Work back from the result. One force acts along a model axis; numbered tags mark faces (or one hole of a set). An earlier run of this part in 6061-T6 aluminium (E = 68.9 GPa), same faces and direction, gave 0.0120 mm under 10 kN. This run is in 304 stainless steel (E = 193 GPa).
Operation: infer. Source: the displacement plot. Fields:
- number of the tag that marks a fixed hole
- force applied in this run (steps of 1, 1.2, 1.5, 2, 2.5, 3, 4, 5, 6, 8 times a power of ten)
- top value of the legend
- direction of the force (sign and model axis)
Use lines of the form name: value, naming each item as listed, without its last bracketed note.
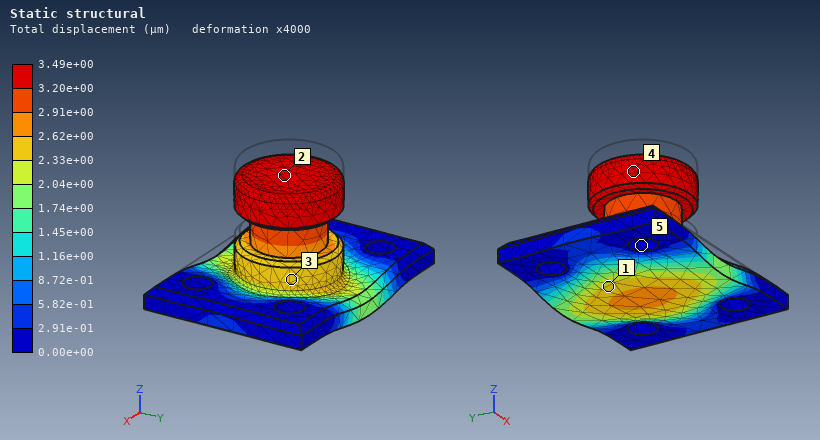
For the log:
number of the tag that marks a fixed hole: 5
force applied in this run: 8 kN
top value of the legend: 3.49e+00 µm
direction of the force: -Z
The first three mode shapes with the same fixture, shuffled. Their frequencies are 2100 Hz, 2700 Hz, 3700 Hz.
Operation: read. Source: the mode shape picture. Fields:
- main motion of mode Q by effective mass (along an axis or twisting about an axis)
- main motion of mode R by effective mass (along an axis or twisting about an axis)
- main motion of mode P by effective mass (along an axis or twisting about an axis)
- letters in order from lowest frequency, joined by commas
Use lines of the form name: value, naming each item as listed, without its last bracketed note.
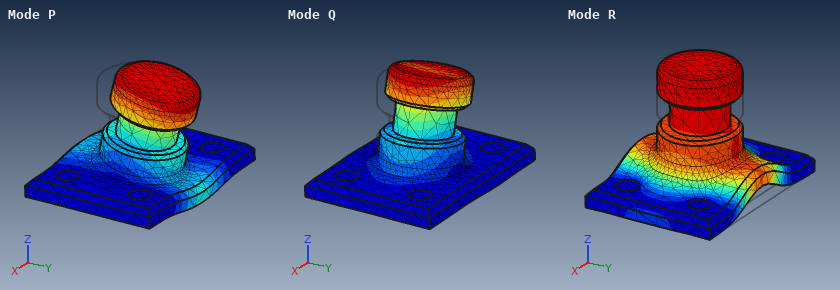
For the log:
main motion of mode Q by effective mass: along X
main motion of mode R by effective mass: along Z
main motion of mode P by effective mass: along Y
letters in order from lowest frequency, joined by commas: P, Q, R
